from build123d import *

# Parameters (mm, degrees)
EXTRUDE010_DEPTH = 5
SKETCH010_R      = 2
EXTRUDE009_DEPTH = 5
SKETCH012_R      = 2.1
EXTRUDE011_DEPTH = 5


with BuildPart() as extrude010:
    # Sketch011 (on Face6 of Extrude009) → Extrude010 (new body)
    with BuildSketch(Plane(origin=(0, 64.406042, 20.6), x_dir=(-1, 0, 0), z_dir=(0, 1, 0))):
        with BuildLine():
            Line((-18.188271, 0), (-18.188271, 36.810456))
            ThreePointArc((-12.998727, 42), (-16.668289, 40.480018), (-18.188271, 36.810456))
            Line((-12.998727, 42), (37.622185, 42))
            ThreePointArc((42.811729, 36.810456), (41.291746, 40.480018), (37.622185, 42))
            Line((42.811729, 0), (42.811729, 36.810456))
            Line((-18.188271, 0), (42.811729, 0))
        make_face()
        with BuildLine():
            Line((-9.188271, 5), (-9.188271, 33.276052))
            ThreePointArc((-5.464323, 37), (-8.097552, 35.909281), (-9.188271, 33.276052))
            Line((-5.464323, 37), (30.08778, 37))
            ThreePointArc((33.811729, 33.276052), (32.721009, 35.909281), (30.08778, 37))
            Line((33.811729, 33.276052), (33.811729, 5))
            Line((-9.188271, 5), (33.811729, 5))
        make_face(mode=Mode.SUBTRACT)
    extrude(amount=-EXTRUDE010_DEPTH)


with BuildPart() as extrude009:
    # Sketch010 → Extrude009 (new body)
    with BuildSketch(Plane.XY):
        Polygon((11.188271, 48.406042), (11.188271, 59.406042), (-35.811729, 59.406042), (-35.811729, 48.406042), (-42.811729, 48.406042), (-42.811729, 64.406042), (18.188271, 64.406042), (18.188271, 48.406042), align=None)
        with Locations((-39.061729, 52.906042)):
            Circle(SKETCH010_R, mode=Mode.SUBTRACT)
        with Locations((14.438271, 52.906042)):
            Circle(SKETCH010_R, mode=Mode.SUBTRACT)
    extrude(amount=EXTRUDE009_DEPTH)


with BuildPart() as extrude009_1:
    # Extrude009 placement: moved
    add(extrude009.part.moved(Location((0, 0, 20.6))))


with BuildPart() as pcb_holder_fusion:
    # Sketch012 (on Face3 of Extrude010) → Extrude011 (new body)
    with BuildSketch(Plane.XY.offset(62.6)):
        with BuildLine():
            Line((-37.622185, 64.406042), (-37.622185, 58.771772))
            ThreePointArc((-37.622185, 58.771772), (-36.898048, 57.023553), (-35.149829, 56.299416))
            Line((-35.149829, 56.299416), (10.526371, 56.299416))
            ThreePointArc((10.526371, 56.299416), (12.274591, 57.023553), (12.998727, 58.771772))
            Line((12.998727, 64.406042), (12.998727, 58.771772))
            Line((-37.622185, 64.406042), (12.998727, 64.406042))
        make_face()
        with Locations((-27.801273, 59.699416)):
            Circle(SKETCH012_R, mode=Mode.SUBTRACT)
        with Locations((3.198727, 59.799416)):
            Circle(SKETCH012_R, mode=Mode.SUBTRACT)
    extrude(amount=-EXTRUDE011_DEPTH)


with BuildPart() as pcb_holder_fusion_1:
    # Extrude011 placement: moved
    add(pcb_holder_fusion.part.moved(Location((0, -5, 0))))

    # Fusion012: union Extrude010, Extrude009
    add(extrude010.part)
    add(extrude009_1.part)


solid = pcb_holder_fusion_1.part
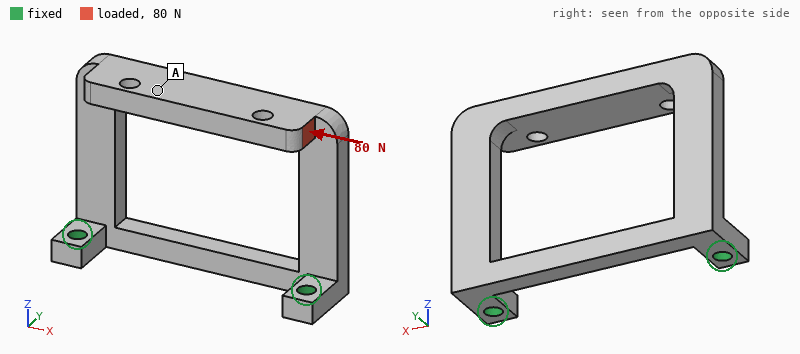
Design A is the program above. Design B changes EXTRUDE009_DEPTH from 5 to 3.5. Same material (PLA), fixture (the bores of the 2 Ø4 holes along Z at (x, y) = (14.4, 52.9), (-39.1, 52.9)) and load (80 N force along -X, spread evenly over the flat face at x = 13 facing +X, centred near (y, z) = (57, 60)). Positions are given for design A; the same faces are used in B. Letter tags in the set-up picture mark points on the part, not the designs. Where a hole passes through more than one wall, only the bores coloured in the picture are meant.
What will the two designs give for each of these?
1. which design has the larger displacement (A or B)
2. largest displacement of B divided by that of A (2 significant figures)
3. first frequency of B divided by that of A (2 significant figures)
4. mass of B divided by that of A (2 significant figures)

B
1.3
0.73
0.98
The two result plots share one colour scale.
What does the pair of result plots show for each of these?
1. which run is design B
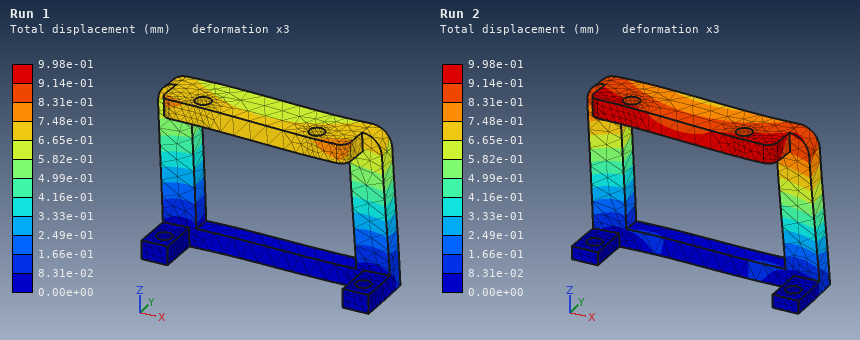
Run 2
